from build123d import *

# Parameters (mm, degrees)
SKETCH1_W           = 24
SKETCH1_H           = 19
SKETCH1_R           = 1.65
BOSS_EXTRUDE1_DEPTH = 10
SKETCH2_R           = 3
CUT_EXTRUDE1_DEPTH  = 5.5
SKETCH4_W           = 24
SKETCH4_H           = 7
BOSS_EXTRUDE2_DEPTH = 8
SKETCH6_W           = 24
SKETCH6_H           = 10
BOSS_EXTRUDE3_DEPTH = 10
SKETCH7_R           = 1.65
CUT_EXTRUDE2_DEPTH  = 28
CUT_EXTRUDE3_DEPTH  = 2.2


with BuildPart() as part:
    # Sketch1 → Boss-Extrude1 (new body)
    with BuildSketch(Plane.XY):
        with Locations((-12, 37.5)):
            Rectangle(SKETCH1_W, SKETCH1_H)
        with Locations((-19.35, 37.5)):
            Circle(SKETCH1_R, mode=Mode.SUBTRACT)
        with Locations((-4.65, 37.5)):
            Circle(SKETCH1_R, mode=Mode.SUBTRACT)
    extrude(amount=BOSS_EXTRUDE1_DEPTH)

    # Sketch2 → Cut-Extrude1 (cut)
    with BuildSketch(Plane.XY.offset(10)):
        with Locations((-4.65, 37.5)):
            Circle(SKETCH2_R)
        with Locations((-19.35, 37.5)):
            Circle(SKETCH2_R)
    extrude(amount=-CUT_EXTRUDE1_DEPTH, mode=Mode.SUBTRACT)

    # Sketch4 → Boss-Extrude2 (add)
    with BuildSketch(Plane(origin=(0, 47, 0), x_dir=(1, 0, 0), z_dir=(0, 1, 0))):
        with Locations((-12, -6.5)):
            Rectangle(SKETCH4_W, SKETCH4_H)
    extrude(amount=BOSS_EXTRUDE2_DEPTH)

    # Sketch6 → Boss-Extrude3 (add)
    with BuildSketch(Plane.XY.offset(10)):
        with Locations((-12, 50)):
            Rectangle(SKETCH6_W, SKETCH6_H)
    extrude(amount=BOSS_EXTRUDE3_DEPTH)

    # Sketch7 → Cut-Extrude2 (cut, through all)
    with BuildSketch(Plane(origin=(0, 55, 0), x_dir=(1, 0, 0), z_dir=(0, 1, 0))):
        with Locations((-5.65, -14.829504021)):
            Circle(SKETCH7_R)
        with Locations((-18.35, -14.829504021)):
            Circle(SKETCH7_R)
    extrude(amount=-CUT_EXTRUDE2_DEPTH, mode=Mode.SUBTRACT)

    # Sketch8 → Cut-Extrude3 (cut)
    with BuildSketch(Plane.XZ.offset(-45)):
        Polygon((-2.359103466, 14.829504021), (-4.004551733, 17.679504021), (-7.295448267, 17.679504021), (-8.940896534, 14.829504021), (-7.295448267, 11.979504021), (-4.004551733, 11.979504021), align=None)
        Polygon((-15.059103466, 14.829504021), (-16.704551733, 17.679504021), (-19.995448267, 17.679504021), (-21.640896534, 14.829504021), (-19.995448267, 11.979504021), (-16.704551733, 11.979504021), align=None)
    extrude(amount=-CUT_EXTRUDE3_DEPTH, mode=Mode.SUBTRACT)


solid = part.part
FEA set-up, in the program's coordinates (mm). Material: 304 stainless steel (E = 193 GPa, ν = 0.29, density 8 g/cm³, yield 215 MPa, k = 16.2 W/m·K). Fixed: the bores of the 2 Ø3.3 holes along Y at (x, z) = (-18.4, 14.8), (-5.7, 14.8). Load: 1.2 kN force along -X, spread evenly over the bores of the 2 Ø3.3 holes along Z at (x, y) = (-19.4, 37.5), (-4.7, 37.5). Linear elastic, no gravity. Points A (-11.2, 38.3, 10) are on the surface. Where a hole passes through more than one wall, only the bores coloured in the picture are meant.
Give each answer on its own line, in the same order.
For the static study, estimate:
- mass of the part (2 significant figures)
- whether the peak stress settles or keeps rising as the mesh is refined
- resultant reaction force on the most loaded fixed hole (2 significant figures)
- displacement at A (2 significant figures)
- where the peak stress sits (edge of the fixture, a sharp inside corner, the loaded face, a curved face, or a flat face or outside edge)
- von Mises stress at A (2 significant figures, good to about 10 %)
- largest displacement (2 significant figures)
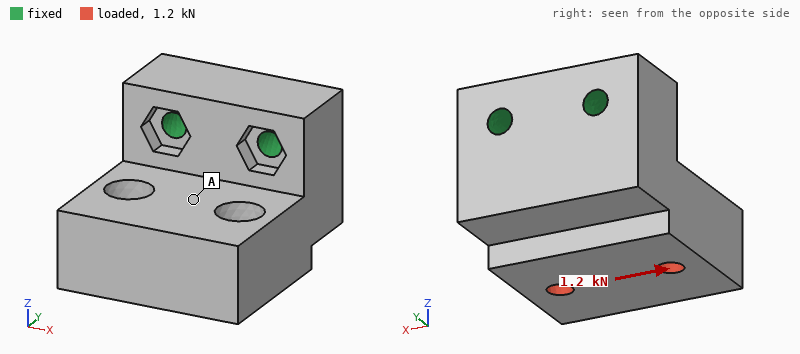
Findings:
61 g
keeps rising
1.5 kN
3.4 µm
edge of the fixture
8.0 MPa
6.8 µm
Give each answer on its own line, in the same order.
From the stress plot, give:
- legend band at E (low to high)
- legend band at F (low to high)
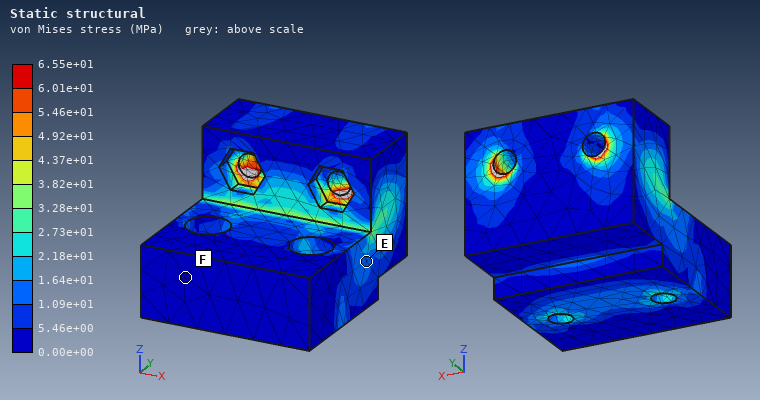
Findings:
1.09e+01 to 1.64e+01 MPa
0.00e+00 to 5.46e+00 MPa
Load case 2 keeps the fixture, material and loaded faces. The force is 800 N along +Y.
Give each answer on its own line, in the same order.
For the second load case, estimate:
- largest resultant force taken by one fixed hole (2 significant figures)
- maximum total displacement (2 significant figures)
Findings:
400 N
8.9 µm
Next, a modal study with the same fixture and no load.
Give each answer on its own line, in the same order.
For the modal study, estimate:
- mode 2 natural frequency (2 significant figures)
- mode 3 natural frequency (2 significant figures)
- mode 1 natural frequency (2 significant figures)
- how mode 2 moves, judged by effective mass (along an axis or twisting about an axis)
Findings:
13 kHz
21 kHz
7900 Hz
along X
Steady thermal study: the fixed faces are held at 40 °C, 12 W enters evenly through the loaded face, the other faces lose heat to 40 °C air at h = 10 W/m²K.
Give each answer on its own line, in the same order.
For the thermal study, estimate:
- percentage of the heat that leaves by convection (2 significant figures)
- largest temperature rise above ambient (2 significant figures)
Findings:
9.2 %
77 K
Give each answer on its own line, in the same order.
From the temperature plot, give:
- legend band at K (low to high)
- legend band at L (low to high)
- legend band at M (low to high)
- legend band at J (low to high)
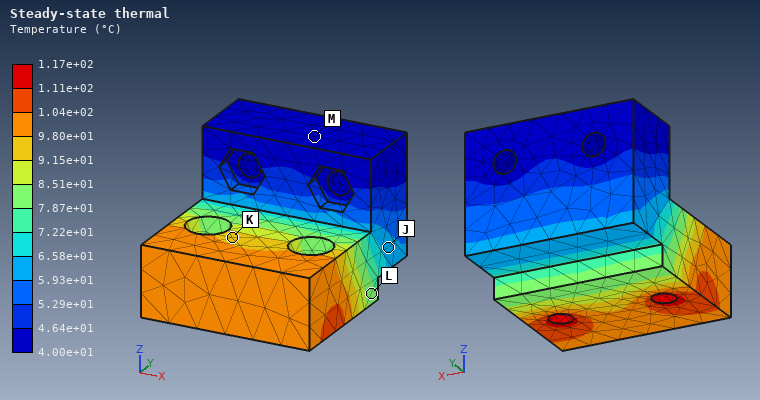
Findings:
9.15e+01 to 9.80e+01 °C
7.87e+01 to 8.51e+01 °C
4.00e+01 to 4.64e+01 °C
5.93e+01 to 6.58e+01 °C
